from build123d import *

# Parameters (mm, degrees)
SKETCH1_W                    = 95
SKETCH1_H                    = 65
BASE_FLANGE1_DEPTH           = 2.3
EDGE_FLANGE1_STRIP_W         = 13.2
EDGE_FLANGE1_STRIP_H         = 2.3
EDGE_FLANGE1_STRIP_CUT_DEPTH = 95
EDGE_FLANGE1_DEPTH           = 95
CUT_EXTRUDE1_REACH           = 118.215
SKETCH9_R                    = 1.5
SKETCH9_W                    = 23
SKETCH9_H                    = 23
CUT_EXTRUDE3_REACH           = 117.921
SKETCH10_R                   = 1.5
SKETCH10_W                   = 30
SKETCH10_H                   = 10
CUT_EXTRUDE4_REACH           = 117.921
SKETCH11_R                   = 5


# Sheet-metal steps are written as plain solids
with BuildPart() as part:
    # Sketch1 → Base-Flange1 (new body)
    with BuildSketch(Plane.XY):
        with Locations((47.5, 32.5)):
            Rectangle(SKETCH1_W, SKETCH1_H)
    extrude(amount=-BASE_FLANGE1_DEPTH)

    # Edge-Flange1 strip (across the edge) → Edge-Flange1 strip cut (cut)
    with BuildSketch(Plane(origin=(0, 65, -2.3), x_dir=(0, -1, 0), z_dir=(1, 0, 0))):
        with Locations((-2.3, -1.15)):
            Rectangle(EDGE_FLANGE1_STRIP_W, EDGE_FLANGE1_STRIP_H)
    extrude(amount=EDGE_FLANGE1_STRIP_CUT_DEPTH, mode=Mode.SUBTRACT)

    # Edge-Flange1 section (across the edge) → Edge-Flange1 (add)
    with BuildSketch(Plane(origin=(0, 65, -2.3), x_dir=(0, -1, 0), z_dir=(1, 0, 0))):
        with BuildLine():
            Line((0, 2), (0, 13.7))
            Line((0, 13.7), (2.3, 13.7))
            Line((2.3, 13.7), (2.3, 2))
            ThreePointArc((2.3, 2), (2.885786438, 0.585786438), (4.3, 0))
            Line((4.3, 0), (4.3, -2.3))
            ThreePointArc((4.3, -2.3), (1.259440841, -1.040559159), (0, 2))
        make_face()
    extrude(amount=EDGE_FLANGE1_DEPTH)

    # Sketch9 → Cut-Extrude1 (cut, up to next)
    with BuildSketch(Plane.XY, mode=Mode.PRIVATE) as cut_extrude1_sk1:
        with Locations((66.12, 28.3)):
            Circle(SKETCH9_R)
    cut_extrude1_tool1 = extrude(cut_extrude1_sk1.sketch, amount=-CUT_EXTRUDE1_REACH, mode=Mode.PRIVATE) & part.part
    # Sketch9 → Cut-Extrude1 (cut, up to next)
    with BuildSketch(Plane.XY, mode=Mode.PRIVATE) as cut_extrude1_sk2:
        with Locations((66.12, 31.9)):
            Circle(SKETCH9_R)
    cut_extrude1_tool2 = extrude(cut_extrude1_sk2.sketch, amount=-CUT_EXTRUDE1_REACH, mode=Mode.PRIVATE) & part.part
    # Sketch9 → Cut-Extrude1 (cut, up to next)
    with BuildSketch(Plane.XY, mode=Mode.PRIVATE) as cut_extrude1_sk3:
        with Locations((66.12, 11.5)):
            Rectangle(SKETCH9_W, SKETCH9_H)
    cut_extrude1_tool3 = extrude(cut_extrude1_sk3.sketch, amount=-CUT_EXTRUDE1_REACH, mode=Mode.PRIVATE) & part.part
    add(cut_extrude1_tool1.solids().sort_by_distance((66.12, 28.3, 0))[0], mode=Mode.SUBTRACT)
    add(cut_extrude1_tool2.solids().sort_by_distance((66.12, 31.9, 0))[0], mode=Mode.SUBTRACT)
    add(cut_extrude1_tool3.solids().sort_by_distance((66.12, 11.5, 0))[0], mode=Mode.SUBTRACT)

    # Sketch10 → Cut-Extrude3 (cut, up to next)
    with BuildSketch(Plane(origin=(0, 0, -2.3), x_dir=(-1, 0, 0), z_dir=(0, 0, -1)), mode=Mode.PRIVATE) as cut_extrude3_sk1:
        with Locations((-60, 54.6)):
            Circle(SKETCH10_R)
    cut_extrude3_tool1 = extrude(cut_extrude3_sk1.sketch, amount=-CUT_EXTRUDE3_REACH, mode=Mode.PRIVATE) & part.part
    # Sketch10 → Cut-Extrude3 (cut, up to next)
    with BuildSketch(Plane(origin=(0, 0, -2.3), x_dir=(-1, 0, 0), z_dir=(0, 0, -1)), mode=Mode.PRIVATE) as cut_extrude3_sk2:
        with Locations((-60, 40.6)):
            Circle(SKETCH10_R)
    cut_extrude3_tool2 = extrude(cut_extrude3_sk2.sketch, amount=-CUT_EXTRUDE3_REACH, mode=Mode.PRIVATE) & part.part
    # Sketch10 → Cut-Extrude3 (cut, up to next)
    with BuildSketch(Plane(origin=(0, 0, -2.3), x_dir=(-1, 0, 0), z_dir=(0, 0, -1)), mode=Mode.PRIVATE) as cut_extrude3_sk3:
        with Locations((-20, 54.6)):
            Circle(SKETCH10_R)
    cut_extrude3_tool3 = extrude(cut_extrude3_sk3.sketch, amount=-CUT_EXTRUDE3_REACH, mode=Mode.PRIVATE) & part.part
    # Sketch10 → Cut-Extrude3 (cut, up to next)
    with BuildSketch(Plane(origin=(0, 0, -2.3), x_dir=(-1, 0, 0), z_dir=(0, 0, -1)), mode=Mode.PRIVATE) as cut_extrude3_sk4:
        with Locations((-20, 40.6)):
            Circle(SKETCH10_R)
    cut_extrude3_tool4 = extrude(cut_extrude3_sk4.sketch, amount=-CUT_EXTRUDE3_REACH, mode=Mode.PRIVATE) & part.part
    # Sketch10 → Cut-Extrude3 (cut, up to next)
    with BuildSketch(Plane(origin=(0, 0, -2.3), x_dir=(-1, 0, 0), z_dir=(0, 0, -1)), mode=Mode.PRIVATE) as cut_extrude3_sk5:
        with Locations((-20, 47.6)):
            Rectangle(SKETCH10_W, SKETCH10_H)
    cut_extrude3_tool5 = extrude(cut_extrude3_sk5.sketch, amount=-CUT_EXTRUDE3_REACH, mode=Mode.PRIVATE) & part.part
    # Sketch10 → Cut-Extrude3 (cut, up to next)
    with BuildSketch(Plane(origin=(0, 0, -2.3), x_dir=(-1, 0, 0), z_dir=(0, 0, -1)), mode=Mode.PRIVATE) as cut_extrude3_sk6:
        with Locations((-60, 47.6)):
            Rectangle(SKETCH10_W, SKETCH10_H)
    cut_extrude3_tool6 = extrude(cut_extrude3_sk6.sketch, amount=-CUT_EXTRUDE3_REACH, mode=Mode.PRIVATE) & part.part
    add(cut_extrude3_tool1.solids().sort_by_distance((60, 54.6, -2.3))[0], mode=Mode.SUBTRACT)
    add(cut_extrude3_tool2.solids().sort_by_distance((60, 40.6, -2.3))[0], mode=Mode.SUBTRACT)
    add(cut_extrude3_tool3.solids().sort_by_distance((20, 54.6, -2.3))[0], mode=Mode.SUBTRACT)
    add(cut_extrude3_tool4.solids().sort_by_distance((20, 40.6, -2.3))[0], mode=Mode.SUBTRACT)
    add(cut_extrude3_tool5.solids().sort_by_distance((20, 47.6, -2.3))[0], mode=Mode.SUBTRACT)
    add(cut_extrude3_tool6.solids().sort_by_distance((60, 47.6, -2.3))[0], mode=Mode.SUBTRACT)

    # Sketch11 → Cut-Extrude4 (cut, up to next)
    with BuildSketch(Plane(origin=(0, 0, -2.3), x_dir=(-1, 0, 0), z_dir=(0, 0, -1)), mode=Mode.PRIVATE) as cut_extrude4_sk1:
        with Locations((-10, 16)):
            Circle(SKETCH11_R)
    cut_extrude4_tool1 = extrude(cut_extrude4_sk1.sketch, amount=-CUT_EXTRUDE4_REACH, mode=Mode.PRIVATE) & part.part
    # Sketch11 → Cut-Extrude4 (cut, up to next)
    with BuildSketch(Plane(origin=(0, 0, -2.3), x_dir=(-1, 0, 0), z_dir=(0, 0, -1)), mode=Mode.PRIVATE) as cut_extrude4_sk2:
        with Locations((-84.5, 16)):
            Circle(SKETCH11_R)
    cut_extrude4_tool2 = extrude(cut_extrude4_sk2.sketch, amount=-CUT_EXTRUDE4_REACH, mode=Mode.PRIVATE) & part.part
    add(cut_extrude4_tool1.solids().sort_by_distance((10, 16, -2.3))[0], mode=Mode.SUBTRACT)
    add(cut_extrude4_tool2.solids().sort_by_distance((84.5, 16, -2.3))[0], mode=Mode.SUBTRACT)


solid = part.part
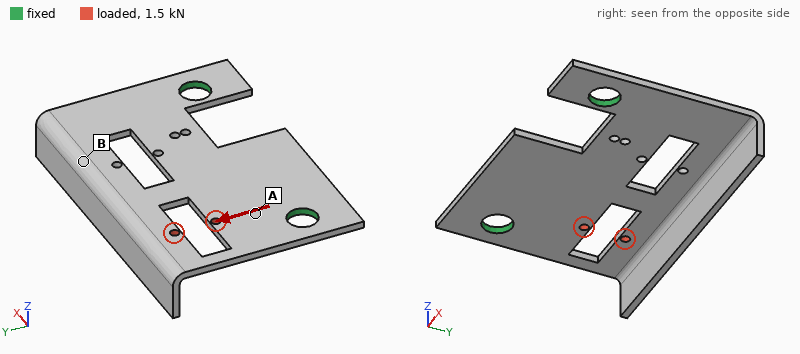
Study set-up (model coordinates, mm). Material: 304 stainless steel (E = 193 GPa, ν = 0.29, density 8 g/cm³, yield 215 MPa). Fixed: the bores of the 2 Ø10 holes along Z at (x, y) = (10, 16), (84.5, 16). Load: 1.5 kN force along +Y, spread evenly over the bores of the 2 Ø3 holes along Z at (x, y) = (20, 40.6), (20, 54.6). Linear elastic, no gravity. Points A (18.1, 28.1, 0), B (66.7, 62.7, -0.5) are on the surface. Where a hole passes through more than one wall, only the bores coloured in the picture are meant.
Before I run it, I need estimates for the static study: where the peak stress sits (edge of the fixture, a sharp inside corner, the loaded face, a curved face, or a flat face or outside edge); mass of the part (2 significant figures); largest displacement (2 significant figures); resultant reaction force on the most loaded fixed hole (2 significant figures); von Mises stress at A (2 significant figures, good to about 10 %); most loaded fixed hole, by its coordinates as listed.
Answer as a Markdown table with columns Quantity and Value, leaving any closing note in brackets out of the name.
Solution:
| Quantity | Value |
|---|---|
| where the peak stress sits | a sharp inside corner |
| mass of the part | 110 g |
| largest displacement | 18 µm |
| resultant reaction force on the most loaded fixed hole | 1.4 kN |
| von Mises stress at A | 25 MPa |
| most loaded fixed hole, by its coordinates as listed | (10, 16) |
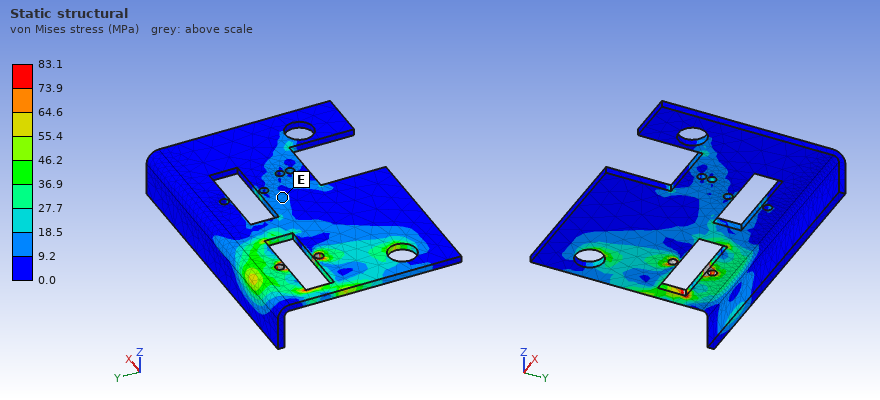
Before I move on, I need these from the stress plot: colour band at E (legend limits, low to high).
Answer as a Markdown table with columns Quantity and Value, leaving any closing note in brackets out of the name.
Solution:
| Quantity | Value |
|---|---|
| colour band at E | 9.2 to 18.5 MPa |
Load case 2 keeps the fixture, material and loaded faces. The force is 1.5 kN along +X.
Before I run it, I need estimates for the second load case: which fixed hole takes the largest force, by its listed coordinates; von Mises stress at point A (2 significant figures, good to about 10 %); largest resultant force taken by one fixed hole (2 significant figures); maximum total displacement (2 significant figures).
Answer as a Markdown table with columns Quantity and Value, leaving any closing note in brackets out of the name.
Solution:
| Quantity | Value |
|---|---|
| which fixed hole takes the largest force, by its listed coordinates | (10, 16) |
| von Mises stress at point A | 22 MPa |
| largest resultant force taken by one fixed hole | 1.2 kN |
| maximum total displacement | 16 µm |
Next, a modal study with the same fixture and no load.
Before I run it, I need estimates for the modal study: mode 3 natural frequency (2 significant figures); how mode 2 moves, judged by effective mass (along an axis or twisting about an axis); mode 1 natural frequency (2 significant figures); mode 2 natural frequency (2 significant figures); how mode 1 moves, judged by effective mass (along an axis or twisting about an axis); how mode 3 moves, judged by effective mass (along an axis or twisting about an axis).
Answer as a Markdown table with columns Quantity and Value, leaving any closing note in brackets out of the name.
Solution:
| Quantity | Value |
|---|---|
| mode 3 natural frequency | 1800 Hz |
| how mode 2 moves, judged by effective mass | twisting about Y |
| mode 1 natural frequency | 460 Hz |
| mode 2 natural frequency | 950 Hz |
| how mode 1 moves, judged by effective mass | along Z |
| how mode 3 moves, judged by effective mass | along Z |
